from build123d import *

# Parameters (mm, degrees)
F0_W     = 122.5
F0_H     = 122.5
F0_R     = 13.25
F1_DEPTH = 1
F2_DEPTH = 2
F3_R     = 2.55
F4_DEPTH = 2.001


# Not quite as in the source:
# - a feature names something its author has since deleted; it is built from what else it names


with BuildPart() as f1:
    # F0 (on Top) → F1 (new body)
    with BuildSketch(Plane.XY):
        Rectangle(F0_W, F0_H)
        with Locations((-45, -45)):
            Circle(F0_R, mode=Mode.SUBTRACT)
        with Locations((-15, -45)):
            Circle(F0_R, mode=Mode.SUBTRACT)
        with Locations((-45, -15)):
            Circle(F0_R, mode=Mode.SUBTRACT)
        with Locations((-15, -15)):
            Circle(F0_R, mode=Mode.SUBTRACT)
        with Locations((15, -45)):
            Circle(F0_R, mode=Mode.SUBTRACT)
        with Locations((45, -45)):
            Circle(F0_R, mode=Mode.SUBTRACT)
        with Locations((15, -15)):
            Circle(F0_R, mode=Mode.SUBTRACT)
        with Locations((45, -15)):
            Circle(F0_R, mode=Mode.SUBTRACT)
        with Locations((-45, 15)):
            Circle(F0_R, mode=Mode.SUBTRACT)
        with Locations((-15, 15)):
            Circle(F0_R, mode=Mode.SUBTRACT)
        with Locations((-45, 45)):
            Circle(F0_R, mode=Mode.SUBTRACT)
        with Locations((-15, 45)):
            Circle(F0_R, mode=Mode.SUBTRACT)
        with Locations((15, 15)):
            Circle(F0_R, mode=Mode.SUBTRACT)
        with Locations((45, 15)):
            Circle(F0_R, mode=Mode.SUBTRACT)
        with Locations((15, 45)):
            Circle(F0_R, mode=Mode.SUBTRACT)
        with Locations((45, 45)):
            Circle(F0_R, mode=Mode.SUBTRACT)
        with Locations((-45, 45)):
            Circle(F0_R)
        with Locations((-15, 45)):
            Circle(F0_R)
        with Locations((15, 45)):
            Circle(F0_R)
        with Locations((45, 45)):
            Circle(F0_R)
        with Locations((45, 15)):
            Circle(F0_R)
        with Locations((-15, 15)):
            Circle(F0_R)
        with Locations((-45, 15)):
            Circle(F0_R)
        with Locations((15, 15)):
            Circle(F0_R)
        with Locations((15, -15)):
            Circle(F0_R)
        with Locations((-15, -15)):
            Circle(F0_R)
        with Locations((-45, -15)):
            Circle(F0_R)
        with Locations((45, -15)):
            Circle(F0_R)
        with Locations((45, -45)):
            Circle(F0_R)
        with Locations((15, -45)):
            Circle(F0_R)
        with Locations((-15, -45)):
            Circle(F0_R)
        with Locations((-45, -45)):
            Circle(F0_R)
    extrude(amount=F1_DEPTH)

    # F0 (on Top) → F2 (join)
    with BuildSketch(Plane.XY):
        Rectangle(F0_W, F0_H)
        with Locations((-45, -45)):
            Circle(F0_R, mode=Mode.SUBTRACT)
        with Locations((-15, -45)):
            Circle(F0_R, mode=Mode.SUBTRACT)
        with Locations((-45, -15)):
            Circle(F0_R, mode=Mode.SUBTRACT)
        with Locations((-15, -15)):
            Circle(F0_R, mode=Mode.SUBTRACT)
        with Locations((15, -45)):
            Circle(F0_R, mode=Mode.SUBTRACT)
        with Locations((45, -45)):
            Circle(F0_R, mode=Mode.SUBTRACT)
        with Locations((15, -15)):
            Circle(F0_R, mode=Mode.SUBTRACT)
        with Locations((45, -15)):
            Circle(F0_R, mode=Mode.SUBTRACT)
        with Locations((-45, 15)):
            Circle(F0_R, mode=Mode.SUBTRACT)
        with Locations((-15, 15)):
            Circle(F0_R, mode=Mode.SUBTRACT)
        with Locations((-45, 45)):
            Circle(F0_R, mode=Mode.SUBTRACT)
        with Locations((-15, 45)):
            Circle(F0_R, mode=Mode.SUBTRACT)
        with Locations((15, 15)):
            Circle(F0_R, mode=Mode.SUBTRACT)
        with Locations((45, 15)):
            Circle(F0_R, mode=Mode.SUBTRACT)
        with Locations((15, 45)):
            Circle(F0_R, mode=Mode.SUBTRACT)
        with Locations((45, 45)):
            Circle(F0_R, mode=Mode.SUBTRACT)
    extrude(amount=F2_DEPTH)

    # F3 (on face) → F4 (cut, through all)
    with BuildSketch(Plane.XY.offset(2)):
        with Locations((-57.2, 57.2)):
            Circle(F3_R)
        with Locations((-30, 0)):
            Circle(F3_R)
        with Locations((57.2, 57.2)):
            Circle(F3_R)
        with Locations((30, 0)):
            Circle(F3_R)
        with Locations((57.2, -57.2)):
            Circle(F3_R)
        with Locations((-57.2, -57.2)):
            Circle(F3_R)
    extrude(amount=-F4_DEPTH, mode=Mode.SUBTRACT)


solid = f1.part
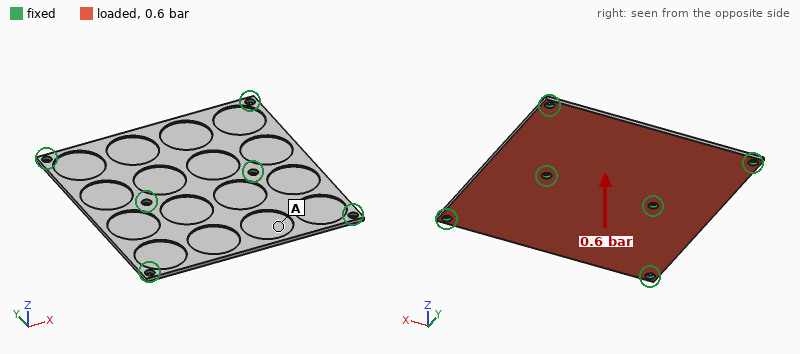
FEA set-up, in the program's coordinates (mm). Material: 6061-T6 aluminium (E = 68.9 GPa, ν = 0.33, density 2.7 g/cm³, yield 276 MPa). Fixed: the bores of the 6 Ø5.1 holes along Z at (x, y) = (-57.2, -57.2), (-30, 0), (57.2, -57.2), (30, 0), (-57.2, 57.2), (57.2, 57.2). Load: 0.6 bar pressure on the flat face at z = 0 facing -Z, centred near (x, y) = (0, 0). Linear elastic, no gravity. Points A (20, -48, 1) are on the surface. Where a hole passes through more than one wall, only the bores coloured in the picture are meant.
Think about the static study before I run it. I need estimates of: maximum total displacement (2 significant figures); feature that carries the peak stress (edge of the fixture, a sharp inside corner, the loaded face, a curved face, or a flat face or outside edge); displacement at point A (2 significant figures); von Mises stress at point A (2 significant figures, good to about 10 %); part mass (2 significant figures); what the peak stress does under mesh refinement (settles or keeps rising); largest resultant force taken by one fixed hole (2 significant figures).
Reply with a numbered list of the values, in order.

1. 0.91 mm
2. edge of the fixture
3. 0.61 mm
4. 24 MPa
5. 57 g
6. keeps rising
7. 260 N
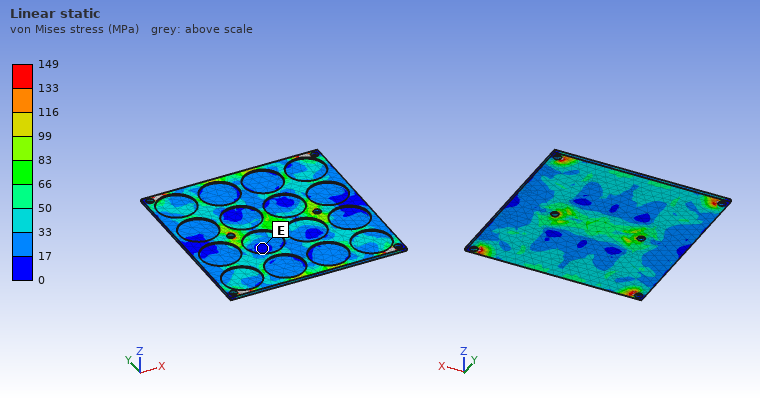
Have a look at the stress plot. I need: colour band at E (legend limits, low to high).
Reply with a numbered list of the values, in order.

1. 0 to 17 MPa
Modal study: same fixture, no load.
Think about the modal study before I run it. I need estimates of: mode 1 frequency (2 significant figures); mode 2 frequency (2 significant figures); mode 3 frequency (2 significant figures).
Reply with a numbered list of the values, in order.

1. 810 Hz
2. 850 Hz
3. 1600 Hz
